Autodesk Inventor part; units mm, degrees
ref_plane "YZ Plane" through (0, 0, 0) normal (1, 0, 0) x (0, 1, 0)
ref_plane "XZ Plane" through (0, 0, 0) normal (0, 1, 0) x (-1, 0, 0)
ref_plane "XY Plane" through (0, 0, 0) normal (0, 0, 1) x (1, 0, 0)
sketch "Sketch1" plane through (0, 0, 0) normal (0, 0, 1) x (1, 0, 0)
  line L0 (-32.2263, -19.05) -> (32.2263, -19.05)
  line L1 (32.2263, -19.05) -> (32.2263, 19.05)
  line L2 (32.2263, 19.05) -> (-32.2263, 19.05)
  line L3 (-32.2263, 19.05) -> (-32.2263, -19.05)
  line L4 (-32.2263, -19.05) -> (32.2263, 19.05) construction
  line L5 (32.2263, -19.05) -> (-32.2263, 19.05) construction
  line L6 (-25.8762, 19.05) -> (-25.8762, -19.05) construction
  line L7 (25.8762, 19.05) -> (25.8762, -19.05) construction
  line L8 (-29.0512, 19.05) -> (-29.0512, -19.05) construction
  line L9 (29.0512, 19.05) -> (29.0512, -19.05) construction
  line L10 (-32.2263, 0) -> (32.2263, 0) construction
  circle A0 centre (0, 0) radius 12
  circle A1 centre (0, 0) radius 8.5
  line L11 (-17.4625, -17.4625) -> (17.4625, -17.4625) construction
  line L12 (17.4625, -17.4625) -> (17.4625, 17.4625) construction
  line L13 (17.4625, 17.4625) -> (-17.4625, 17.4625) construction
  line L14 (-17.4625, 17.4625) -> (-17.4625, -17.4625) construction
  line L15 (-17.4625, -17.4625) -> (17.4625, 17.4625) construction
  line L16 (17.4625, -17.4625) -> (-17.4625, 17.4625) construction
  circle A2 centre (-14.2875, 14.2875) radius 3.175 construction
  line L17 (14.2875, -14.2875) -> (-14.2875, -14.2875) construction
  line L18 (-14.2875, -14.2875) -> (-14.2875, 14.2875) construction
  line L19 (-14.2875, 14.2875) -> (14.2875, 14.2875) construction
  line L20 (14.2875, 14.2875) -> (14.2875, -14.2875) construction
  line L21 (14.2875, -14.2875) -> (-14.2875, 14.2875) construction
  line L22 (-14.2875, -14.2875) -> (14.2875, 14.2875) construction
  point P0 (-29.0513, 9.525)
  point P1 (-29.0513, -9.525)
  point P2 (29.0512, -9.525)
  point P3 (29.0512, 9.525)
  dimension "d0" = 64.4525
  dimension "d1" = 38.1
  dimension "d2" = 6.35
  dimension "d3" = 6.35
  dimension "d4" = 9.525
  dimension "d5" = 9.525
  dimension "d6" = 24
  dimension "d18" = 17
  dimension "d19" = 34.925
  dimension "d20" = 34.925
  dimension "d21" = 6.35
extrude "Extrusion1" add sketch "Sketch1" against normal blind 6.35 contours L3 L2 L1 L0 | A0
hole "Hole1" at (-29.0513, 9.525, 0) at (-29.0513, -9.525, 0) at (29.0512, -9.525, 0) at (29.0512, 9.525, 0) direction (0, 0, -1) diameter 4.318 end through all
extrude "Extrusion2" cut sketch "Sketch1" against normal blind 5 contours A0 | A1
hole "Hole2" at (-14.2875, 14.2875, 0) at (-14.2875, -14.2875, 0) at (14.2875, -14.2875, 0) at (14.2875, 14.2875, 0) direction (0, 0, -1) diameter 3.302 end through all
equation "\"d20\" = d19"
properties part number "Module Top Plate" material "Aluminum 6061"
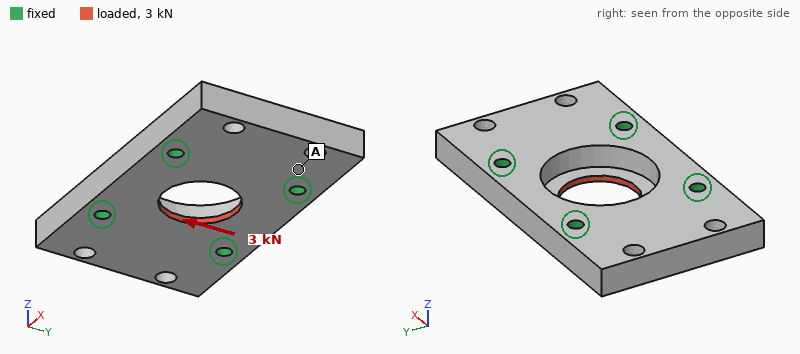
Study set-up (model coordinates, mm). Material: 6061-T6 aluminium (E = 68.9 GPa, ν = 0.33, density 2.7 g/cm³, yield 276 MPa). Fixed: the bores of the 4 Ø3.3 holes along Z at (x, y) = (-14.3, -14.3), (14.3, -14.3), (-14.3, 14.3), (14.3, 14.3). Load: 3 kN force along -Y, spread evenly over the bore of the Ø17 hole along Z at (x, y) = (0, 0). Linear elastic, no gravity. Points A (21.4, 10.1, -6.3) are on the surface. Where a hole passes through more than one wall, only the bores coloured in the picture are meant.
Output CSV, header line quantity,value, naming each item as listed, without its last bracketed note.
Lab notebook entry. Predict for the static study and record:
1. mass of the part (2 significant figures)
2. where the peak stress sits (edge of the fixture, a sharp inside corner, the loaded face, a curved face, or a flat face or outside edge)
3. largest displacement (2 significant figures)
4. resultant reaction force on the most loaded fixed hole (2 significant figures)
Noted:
quantity,value
mass of the part,34 g
where the peak stress sits,a sharp inside corner
largest displacement,12 µm
resultant reaction force on the most loaded fixed hole,790 N
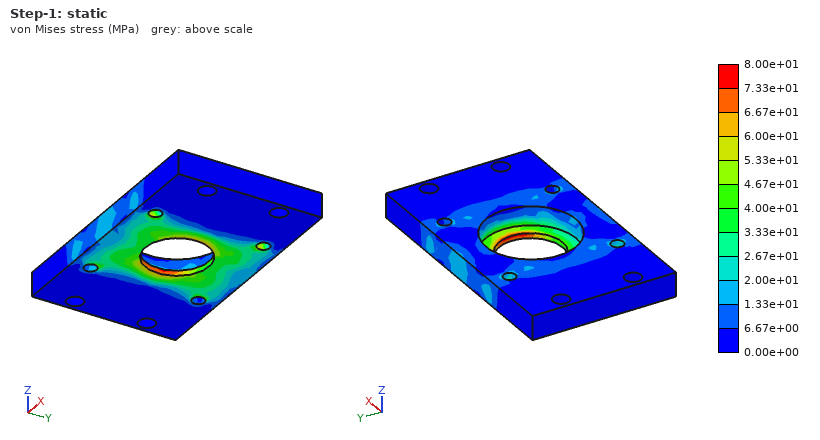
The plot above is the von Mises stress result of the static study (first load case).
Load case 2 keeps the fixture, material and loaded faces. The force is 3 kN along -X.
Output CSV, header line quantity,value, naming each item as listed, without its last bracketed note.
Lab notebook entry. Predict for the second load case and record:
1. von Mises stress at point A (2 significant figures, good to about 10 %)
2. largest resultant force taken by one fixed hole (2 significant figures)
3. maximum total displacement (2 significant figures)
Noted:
quantity,value
von Mises stress at point A,8.8 MPa
largest resultant force taken by one fixed hole,760 N
maximum total displacement,9.6 µm
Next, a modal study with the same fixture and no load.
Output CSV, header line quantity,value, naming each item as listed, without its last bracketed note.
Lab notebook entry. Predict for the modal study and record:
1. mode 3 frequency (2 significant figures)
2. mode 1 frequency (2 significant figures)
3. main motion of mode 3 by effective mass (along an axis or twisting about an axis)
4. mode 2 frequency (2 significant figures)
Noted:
quantity,value
mode 3 frequency,21 kHz
mode 1 frequency,12 kHz
main motion of mode 3 by effective mass,twisting about X
mode 2 frequency,13 kHz
